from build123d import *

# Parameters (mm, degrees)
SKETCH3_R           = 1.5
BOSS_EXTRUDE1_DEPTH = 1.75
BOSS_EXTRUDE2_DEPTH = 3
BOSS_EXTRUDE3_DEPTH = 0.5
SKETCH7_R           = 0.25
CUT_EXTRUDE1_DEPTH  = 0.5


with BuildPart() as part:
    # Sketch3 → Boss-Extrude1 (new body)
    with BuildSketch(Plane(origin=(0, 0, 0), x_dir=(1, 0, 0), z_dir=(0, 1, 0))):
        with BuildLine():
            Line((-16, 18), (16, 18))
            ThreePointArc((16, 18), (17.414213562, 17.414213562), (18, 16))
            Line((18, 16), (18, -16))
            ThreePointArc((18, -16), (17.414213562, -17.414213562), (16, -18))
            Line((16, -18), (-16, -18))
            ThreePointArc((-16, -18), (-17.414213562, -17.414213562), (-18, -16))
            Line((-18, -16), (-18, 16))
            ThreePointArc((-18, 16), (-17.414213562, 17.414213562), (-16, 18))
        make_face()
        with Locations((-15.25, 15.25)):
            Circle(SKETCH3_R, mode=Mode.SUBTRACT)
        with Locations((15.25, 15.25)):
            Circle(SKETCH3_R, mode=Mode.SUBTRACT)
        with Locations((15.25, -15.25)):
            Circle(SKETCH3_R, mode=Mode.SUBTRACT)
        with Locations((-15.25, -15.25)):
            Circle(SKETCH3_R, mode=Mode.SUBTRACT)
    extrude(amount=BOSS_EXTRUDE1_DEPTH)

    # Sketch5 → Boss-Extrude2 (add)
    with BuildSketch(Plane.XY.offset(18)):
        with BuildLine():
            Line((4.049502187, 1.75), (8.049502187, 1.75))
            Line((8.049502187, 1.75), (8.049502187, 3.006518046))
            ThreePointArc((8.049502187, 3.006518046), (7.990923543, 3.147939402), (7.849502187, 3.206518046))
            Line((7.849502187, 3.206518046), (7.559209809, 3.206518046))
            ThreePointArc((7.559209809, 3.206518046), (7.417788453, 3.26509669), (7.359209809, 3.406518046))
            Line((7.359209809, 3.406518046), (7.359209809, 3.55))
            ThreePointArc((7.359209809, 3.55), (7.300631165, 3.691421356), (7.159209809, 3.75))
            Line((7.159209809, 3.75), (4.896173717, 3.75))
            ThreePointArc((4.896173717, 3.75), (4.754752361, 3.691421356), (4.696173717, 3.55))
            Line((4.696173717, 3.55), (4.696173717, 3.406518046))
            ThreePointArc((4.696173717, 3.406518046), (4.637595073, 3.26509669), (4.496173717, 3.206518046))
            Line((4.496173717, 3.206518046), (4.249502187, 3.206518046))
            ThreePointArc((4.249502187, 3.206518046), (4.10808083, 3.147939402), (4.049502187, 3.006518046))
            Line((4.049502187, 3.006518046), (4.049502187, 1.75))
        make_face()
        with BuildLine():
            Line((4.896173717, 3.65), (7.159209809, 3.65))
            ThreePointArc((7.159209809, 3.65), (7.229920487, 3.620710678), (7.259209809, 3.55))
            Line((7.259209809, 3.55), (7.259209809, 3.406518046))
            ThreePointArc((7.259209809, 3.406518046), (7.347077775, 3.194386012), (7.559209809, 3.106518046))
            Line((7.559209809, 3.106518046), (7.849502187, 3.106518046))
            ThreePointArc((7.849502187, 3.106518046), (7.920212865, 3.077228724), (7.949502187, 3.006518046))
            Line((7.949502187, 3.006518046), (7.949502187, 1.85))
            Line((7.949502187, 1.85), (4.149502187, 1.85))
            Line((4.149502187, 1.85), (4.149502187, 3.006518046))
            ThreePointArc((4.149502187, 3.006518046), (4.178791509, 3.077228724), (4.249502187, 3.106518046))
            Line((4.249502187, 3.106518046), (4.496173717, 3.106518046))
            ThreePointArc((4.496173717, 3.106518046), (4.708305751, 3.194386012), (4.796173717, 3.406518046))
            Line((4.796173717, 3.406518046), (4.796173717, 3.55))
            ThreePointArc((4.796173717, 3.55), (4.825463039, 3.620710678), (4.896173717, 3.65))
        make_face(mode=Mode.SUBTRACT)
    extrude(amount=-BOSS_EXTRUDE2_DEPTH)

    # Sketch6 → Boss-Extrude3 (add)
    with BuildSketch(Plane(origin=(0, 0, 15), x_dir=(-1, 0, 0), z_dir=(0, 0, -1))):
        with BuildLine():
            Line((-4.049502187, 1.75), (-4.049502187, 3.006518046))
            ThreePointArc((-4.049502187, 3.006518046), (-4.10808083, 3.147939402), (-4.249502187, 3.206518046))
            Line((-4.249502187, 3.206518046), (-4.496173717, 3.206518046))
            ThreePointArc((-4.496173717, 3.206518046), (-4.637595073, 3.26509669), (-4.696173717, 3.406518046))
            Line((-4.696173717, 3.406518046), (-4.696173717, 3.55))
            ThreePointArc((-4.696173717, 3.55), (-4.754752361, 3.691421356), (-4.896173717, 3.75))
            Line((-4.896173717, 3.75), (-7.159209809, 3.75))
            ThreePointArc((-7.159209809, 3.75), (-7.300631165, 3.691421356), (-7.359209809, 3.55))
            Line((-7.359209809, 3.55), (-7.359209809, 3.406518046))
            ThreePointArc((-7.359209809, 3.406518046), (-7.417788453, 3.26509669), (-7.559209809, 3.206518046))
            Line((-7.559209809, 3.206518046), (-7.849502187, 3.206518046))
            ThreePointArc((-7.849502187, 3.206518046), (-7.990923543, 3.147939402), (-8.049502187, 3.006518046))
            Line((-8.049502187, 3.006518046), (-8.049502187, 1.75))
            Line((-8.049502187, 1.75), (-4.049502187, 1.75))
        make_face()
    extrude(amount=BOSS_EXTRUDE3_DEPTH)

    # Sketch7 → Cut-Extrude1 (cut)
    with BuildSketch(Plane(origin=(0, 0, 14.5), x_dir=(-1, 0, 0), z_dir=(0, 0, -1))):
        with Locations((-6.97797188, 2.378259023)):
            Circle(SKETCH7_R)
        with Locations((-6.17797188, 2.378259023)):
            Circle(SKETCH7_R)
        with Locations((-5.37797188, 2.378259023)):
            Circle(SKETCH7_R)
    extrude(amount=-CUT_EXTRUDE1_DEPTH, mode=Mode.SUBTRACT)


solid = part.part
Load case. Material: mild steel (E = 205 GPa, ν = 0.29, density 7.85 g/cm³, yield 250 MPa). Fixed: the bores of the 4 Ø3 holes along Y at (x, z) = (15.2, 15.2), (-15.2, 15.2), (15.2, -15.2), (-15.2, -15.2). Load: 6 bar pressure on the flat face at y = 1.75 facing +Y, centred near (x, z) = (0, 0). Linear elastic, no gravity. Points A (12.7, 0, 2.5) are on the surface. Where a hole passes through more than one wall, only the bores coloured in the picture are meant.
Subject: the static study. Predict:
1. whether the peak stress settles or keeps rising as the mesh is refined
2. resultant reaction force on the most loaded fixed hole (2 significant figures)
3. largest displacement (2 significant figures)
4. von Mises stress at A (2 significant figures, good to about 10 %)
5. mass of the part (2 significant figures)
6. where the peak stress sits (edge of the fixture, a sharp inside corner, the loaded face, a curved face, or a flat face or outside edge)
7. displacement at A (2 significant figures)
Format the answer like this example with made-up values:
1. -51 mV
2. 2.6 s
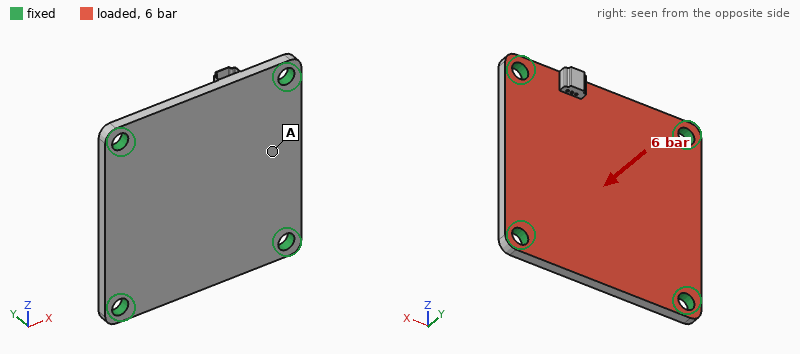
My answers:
1. keeps rising
2. 190 N
3. 34 µm
4. 49 MPa
5. 17 g
6. edge of the fixture
7. 20 µm
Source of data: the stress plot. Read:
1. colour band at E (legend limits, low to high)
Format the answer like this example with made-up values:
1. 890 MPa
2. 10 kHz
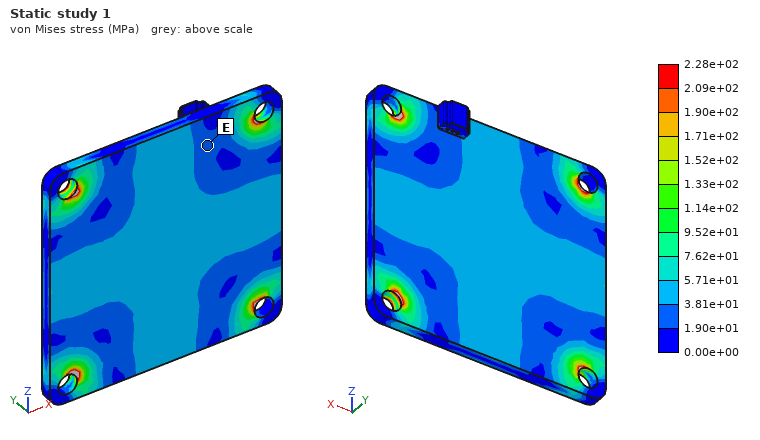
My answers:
1. 1.90e+01 to 3.81e+01 MPa
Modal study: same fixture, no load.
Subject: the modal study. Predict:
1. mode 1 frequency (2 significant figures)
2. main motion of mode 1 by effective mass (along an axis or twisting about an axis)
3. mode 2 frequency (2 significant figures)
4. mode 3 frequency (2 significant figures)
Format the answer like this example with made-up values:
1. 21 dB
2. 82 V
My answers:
1. 7000 Hz
2. along Y
3. 12 kHz
4. 12 kHz
